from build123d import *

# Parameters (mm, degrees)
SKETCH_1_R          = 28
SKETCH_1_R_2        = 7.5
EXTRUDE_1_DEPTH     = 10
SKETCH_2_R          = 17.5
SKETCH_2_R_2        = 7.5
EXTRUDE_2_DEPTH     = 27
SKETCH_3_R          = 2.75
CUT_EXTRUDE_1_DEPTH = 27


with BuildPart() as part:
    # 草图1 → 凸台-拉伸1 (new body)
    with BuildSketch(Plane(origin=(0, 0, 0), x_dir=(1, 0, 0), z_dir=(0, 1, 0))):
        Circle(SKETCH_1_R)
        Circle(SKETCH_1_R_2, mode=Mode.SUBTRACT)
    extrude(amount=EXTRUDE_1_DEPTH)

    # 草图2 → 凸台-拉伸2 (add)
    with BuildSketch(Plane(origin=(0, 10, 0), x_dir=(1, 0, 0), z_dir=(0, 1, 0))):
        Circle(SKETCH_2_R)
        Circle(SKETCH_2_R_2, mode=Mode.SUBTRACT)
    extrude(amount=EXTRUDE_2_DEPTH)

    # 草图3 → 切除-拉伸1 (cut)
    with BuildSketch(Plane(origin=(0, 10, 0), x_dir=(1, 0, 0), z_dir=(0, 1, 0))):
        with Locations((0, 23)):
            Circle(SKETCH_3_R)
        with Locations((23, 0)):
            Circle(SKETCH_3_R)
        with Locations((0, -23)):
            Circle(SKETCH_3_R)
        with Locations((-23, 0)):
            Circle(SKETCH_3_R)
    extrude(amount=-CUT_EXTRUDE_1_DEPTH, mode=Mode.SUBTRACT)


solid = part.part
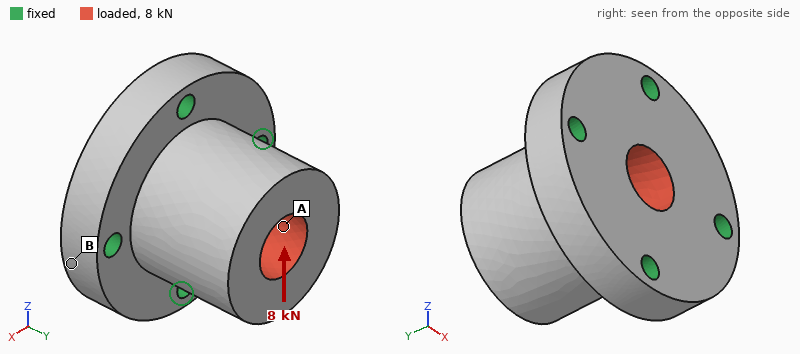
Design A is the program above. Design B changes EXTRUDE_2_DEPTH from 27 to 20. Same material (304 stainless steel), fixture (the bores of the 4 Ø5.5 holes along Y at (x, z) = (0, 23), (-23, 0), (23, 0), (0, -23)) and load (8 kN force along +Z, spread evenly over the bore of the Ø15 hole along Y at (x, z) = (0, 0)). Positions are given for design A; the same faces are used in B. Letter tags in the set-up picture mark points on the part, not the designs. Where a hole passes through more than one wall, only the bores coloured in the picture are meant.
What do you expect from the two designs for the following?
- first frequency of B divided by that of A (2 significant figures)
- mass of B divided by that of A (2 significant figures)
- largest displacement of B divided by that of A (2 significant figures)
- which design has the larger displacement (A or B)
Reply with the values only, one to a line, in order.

1.4
0.87
0.63
A
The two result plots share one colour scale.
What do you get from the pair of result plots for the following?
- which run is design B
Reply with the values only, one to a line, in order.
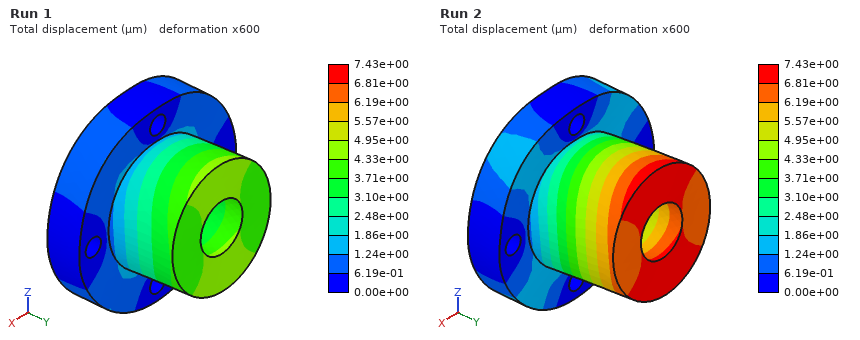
Run 1
